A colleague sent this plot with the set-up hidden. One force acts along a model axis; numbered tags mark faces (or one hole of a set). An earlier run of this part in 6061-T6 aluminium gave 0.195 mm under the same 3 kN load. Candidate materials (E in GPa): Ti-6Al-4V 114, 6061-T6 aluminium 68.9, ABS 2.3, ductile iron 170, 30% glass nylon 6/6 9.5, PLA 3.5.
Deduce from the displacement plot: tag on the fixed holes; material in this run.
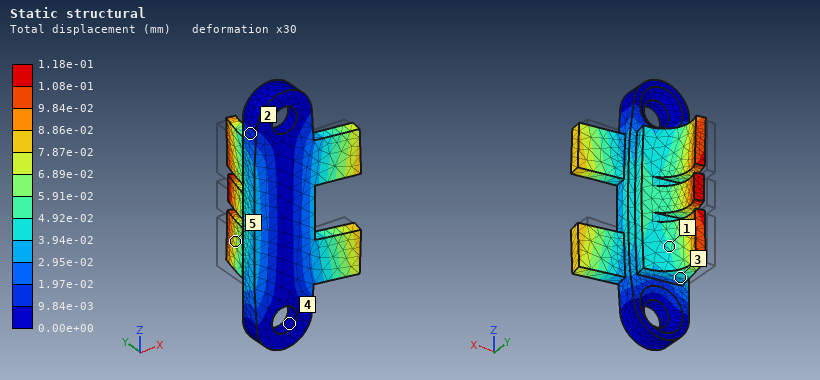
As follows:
4
Ti-6Al-4V
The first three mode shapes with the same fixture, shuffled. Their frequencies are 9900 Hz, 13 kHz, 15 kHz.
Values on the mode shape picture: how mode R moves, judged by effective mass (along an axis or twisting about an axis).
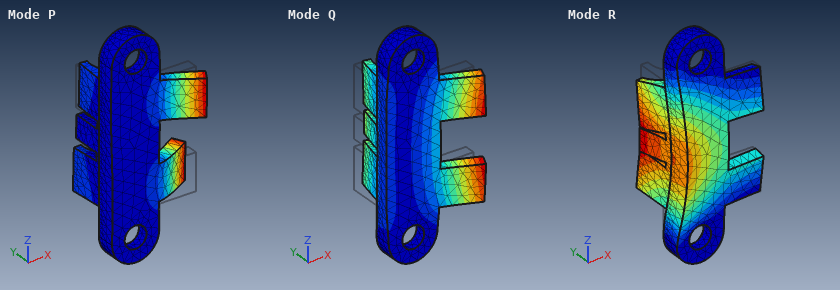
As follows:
along Y
